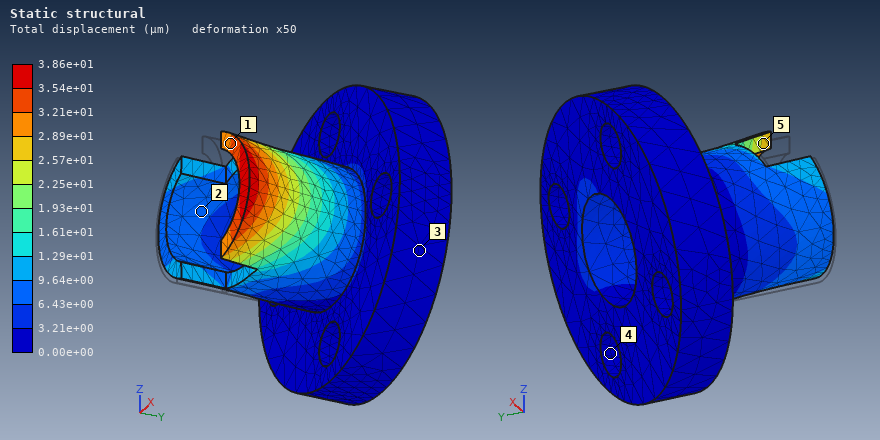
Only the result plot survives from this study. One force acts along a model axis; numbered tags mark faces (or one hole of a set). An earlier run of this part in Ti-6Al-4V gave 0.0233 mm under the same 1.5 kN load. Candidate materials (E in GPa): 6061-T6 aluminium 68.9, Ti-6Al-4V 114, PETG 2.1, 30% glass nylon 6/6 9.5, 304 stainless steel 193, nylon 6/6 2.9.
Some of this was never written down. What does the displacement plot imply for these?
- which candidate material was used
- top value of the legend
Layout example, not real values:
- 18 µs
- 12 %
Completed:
- 6061-T6 aluminium
- 3.86e+01 µm
